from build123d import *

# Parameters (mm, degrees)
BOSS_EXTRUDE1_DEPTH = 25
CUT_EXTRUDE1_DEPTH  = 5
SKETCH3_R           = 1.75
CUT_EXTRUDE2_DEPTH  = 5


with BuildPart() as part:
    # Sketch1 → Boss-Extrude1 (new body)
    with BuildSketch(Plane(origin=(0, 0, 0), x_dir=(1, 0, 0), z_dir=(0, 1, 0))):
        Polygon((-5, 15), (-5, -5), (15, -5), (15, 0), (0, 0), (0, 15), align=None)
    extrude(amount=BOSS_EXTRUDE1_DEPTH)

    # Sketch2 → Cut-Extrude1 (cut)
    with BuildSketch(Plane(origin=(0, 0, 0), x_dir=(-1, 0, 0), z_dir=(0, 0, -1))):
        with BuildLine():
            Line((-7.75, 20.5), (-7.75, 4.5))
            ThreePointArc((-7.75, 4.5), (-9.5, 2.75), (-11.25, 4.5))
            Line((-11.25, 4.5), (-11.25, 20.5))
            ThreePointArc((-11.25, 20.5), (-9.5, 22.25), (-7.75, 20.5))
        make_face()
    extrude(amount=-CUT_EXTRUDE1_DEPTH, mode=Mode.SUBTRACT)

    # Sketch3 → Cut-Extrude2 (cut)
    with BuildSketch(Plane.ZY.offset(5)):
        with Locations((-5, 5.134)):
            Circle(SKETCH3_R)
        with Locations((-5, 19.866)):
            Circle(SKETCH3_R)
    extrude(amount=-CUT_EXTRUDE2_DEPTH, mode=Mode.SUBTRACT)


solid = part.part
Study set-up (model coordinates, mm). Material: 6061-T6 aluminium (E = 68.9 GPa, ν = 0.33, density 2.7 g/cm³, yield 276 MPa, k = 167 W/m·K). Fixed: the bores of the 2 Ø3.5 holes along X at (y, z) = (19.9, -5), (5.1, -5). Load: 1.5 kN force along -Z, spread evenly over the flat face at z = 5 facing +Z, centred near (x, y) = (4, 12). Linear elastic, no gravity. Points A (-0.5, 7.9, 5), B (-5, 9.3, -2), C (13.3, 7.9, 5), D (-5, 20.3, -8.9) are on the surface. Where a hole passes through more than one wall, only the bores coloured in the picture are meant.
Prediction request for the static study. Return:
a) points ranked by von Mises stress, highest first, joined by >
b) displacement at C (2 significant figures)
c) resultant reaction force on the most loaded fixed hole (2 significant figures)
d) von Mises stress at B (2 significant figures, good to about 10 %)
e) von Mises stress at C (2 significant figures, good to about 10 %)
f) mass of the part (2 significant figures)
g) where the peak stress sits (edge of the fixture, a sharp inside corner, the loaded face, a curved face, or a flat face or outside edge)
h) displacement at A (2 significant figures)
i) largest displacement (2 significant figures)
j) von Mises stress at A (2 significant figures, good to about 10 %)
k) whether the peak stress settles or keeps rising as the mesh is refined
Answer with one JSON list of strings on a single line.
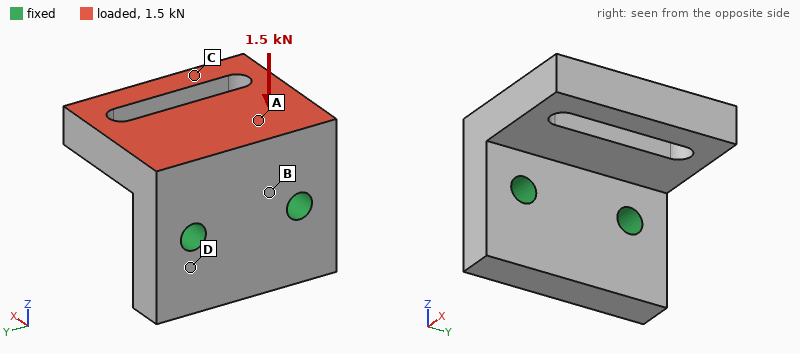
["B > A > C > D", "0.12 mm", "760 N", "64 MPa", "24 MPa", "11 g", "edge of the fixture", "0.028 mm", "0.13 mm", "51 MPa", "keeps rising"]
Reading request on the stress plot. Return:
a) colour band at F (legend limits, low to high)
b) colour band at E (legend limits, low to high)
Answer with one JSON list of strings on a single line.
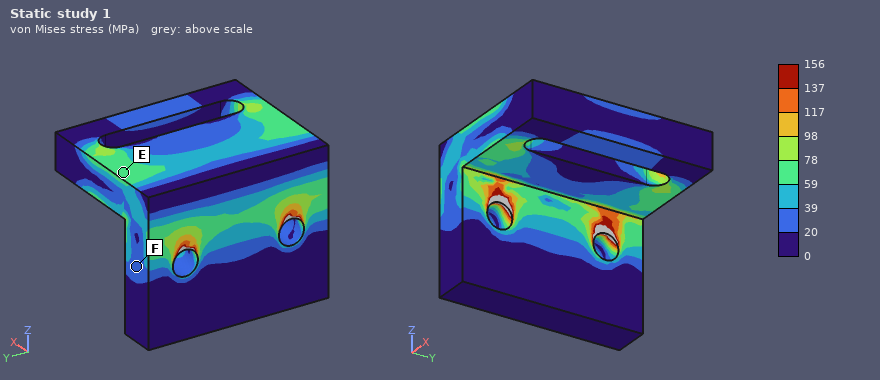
["20 to 39 MPa", "59 to 78 MPa"]
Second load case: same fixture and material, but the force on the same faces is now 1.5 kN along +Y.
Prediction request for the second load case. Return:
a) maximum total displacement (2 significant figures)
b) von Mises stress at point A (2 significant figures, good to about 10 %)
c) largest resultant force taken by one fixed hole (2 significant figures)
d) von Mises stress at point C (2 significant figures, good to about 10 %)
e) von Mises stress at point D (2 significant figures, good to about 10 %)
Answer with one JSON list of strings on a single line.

["35 µm", "14 MPa", "1.3 kN", "16 MPa", "11 MPa"]
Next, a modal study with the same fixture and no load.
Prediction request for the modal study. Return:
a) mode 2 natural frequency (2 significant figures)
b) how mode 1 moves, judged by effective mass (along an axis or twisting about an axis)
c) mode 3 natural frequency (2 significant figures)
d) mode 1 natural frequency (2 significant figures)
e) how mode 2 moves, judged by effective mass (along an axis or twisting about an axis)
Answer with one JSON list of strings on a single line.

["15 kHz", "along Z", "19 kHz", "8400 Hz", "along Y"]
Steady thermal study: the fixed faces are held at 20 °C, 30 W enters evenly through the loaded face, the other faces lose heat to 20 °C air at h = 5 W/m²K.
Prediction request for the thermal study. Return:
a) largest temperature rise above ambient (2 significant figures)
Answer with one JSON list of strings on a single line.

["30 K"]
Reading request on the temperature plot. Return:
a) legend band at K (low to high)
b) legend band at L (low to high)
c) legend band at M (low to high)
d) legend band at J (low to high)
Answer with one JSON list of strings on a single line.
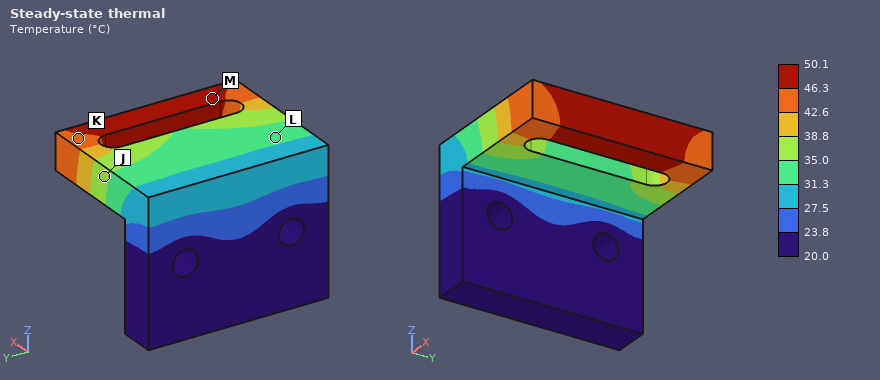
["42.6 to 46.3 °C", "31.3 to 35.0 °C", "46.3 to 50.1 °C", "35.0 to 38.8 °C"]
